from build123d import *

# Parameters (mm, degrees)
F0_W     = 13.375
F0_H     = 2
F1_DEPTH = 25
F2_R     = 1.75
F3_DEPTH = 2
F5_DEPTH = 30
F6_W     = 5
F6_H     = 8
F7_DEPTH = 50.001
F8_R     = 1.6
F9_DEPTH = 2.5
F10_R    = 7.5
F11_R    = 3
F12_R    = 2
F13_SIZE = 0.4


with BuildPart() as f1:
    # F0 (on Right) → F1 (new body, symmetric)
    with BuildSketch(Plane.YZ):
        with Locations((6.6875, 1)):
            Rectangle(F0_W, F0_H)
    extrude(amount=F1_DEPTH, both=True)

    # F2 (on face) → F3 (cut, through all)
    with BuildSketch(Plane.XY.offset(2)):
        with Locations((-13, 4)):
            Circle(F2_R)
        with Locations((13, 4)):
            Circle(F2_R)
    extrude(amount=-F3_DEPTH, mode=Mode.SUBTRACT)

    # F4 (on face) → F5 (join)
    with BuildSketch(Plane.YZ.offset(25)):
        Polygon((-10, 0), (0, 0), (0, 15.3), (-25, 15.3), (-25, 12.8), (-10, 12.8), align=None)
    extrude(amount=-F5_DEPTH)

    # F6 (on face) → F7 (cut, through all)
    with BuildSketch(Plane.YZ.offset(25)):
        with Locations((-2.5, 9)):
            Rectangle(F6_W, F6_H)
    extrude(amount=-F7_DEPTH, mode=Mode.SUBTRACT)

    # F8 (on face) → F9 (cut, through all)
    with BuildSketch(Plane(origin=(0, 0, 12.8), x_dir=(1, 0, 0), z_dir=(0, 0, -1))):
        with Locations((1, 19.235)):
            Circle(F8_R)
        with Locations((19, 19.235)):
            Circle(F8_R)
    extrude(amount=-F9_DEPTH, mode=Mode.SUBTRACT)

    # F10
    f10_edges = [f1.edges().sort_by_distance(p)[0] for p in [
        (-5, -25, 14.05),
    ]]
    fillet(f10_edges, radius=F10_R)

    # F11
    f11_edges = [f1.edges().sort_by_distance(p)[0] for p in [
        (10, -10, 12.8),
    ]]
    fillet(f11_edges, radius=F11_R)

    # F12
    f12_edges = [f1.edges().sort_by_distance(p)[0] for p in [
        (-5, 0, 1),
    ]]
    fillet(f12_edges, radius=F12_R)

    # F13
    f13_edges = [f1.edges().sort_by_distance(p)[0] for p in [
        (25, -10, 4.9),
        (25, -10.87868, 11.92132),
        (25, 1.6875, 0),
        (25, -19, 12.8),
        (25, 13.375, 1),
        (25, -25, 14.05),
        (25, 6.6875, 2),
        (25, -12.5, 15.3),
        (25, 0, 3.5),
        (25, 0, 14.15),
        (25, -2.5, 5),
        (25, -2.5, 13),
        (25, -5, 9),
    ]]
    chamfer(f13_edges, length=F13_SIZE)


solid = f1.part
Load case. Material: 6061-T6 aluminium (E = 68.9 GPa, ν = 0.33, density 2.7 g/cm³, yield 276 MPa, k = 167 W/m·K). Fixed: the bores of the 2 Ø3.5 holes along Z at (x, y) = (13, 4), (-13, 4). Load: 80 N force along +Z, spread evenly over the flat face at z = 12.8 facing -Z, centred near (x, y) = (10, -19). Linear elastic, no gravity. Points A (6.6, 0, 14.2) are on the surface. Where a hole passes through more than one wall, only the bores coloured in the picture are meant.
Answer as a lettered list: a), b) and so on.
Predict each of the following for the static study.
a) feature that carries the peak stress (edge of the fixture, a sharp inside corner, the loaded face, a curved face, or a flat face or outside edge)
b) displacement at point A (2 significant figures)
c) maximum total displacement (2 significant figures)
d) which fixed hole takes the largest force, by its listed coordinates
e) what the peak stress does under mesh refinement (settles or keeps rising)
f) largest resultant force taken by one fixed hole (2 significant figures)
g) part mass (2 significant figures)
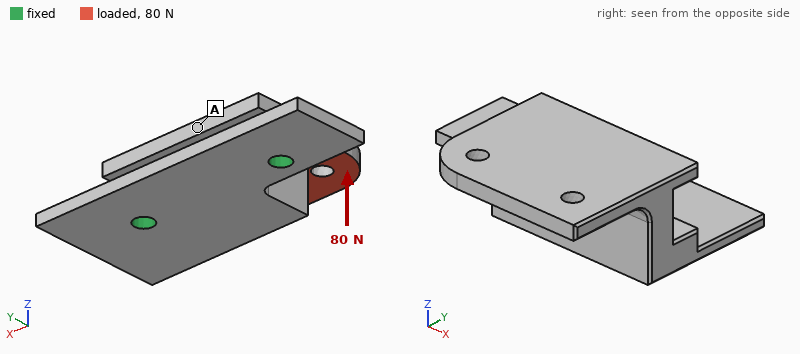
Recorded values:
a) edge of the fixture
b) 0.086 mm
c) 0.21 mm
d) (13, 4)
e) keeps rising
f) 75 N
g) 16 g
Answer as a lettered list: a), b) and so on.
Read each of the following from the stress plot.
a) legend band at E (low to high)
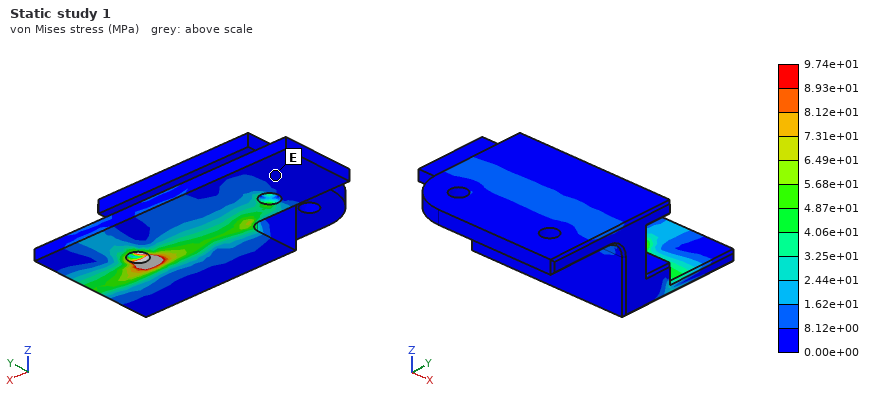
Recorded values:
a) 0.00e+00 to 8.12e+00 MPa
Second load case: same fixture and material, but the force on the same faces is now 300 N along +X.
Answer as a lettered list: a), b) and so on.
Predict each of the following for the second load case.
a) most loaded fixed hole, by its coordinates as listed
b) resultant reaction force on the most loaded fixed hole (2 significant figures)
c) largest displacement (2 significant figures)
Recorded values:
a) (13, 4)
b) 350 N
c) 53 µm
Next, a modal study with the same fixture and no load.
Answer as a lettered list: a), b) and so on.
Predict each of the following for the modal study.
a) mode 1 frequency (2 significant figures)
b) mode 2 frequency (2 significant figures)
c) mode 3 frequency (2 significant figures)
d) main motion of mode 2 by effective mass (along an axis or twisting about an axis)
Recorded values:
a) 1500 Hz
b) 4300 Hz
c) 8200 Hz
d) along X
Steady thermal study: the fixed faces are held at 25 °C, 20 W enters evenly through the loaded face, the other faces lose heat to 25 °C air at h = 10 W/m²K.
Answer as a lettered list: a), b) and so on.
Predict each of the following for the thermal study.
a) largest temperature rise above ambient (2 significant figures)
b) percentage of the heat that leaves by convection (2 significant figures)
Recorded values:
a) 43 K
b) 3.7 %
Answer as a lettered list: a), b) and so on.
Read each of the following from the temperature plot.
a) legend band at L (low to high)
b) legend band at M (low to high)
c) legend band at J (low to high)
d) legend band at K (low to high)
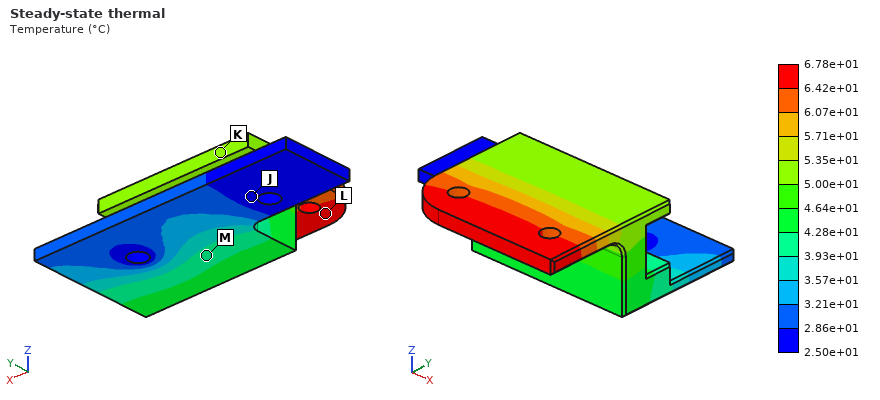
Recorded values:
a) 6.42e+01 to 6.78e+01 °C
b) 3.93e+01 to 4.28e+01 °C
c) 2.50e+01 to 2.86e+01 °C
d) 5.00e+01 to 5.35e+01 °C
